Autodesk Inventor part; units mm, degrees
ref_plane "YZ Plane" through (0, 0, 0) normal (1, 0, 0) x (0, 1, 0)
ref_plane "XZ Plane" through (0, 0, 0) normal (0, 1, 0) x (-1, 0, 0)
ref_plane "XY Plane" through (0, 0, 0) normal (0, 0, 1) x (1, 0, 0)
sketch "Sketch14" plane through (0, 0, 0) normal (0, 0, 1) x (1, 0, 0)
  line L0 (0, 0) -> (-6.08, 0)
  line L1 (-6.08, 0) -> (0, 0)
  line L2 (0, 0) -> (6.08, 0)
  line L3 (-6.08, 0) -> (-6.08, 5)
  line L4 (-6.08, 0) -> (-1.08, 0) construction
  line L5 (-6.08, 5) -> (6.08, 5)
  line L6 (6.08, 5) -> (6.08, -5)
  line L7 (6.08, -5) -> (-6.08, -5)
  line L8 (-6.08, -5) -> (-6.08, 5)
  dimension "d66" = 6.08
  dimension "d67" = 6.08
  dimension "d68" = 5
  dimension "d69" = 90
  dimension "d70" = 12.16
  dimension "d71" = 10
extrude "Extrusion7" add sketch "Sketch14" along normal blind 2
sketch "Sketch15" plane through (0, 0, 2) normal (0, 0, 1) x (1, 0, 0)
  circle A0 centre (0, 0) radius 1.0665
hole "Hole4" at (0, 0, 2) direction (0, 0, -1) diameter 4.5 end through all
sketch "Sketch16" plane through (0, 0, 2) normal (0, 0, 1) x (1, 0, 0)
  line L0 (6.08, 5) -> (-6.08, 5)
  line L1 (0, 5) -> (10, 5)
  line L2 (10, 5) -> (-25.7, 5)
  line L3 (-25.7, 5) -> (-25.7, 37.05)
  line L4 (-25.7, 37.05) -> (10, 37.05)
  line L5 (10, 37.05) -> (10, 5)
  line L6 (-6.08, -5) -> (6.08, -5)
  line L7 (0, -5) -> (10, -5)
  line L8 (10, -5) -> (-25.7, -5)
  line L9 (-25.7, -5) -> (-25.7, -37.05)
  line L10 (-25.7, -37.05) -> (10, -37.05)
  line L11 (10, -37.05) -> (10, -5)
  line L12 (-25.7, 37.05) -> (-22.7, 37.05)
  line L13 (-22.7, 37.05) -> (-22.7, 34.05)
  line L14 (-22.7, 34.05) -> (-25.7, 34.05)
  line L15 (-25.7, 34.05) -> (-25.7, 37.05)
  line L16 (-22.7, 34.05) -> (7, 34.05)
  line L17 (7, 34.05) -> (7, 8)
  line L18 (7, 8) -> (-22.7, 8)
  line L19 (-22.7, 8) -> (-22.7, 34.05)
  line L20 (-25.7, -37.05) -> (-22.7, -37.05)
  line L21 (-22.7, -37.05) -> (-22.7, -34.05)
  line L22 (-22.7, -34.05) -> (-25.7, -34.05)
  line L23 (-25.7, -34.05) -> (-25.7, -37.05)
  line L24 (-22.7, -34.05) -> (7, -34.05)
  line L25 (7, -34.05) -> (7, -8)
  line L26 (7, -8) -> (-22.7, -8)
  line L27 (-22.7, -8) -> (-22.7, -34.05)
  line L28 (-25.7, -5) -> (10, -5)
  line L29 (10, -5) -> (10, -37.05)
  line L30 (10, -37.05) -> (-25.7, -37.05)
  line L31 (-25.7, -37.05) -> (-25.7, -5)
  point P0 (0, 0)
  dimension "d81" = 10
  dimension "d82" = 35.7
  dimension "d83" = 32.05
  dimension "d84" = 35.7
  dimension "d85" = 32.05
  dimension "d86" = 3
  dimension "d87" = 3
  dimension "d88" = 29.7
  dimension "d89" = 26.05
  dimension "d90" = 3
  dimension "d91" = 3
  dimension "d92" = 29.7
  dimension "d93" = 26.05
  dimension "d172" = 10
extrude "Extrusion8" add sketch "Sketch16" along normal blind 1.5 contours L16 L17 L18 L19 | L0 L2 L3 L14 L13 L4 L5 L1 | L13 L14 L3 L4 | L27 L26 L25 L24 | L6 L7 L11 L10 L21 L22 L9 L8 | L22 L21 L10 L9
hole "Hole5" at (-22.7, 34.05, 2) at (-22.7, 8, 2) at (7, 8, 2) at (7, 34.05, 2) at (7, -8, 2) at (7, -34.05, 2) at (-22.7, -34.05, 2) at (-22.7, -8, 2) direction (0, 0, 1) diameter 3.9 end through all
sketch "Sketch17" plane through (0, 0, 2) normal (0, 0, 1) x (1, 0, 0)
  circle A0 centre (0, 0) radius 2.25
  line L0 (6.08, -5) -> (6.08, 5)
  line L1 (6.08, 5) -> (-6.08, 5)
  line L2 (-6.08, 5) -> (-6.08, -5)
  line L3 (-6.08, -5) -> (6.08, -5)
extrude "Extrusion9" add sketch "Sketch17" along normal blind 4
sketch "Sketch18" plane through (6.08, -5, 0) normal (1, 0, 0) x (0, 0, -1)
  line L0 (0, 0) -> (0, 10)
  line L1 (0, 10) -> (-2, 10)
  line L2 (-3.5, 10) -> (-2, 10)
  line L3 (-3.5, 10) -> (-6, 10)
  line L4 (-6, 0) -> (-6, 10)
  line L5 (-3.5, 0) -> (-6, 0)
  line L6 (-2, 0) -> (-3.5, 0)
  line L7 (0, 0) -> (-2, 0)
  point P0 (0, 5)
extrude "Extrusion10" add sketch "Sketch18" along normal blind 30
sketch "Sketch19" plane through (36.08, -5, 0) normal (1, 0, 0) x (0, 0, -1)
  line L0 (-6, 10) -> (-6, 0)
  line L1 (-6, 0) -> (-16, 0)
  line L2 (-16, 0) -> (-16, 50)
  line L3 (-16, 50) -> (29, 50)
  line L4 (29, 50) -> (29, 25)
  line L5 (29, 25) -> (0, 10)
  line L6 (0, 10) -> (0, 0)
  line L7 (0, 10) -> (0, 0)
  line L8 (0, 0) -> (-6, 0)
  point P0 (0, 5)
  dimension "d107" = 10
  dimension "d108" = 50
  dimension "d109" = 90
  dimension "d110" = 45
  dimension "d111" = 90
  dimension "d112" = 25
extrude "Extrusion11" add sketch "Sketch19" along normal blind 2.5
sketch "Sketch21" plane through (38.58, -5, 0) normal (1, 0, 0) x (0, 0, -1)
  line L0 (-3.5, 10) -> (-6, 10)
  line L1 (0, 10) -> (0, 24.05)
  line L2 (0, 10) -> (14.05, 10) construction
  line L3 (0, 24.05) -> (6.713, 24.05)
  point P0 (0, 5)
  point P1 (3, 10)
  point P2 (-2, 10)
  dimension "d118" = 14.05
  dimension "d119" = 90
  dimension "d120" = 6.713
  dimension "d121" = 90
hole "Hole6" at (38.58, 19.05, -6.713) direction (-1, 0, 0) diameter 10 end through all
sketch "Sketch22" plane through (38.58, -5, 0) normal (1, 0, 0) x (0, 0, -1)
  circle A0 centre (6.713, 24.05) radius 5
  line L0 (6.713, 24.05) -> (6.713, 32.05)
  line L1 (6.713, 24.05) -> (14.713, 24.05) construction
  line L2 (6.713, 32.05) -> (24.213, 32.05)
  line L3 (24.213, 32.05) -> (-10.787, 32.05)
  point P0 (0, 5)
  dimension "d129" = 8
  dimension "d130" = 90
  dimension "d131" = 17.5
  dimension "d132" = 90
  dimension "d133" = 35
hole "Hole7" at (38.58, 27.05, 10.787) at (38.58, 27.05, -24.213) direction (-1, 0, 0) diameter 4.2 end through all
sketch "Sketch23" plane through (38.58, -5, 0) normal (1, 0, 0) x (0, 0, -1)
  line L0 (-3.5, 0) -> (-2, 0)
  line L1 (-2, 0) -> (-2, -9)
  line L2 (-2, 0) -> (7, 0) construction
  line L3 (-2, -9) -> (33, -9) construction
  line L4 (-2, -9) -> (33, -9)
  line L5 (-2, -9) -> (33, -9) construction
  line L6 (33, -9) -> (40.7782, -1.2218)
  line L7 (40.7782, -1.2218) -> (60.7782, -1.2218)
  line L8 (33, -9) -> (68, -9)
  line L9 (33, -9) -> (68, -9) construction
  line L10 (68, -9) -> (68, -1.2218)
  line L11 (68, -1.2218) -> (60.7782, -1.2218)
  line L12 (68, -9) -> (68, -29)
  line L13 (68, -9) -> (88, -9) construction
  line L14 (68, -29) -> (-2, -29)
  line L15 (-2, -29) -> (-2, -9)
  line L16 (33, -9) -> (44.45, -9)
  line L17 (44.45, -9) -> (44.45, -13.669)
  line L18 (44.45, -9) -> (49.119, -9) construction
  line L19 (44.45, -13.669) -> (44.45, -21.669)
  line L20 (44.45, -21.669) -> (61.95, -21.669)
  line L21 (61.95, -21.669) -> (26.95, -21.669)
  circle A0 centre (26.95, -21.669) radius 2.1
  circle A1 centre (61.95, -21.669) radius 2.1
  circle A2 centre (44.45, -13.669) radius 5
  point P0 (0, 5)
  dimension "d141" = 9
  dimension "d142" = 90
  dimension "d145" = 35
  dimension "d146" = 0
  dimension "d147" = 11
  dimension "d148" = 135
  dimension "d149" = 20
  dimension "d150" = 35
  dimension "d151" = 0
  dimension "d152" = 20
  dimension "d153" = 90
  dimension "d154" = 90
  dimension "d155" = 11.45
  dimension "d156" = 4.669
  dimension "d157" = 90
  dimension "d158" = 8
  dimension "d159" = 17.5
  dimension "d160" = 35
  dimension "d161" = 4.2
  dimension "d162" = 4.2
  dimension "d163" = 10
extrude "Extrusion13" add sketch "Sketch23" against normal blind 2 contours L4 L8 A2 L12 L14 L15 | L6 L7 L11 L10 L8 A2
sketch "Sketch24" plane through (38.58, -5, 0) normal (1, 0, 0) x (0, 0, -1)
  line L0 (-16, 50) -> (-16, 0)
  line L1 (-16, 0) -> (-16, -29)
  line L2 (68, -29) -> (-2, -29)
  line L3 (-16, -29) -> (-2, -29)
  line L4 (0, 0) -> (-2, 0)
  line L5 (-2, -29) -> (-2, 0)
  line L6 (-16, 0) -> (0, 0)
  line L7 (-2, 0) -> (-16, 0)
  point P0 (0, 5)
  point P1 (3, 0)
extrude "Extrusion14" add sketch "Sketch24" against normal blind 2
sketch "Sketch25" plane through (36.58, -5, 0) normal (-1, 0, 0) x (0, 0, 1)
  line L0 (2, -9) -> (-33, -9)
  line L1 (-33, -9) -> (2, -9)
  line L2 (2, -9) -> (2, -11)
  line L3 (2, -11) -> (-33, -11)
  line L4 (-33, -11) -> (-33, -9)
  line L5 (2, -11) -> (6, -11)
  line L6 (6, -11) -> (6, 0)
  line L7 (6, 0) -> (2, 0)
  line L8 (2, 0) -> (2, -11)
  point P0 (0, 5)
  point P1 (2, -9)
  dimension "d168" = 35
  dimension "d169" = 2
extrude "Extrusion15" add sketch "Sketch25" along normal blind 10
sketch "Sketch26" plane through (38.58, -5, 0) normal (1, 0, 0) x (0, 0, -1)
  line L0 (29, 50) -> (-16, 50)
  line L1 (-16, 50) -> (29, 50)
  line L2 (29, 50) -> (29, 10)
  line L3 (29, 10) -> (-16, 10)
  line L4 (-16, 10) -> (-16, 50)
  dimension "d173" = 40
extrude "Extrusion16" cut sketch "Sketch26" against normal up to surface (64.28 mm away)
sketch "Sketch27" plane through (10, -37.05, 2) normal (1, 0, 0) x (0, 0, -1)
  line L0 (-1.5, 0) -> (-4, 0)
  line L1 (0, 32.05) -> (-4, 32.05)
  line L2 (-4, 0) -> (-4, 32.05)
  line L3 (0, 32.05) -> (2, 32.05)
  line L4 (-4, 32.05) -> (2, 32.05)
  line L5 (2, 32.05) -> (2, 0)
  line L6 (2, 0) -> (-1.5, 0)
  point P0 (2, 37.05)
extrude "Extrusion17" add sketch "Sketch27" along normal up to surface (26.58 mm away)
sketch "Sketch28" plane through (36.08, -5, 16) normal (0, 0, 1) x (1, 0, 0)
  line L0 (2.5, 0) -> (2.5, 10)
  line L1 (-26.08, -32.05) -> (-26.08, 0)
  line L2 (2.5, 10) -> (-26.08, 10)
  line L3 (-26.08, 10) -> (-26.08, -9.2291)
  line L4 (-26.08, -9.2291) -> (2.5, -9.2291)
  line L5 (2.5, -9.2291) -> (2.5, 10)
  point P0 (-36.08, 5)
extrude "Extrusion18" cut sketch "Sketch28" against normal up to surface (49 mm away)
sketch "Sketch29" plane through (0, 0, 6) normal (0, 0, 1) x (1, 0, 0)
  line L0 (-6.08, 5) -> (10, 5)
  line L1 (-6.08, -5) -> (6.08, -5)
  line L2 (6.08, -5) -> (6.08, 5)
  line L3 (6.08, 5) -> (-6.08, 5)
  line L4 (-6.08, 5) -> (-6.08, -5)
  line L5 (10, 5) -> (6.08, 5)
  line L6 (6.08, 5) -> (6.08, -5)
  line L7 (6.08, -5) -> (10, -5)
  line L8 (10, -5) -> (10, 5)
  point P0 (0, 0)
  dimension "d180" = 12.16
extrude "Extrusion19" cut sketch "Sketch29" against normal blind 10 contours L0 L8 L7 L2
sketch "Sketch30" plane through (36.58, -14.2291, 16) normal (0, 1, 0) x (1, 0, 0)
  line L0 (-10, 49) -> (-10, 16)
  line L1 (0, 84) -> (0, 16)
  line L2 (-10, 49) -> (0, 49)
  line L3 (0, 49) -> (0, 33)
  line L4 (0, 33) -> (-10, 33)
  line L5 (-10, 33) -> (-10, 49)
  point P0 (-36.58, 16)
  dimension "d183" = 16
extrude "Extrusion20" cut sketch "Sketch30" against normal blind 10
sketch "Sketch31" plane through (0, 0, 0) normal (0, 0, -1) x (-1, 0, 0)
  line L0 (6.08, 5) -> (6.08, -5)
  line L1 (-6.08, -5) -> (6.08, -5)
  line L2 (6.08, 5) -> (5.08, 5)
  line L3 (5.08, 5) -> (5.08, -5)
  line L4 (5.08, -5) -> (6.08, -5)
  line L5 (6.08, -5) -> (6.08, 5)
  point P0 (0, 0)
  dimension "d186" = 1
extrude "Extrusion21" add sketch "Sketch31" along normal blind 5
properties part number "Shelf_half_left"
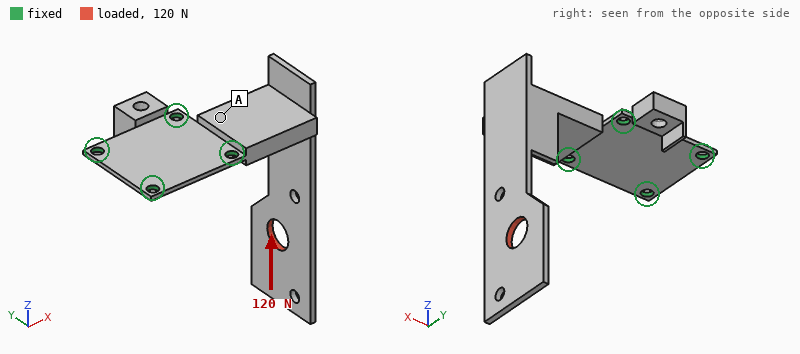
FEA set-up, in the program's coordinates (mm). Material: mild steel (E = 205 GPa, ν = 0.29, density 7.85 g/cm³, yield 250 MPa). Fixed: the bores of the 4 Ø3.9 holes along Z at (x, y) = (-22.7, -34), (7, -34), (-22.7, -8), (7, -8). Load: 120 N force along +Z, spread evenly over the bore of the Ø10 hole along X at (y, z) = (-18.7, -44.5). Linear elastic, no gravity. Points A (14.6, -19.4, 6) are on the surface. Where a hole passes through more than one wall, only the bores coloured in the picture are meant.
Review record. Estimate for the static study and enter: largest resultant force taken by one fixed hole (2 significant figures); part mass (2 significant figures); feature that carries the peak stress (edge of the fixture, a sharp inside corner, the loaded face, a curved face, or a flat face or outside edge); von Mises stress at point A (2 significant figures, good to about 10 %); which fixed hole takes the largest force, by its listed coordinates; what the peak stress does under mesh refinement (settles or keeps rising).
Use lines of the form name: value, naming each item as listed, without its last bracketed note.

largest resultant force taken by one fixed hole: 92 N
part mass: 78 g
feature that carries the peak stress: edge of the fixture
von Mises stress at point A: 27 MPa
which fixed hole takes the largest force, by its listed coordinates: (7, -8)
what the peak stress does under mesh refinement: keeps rising
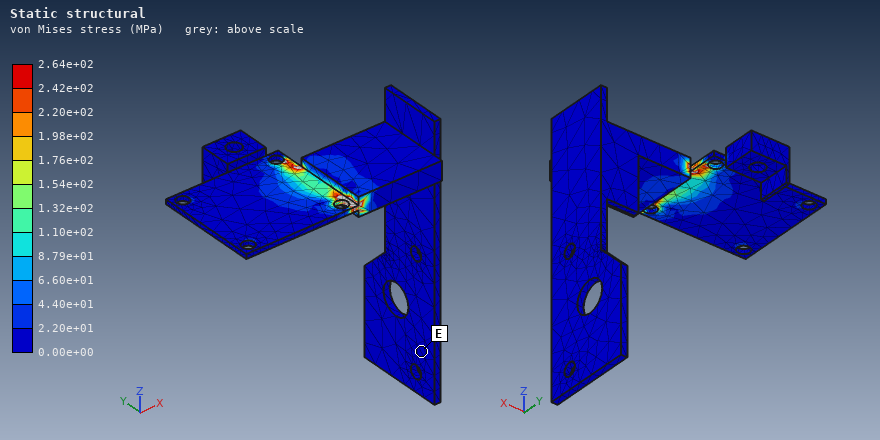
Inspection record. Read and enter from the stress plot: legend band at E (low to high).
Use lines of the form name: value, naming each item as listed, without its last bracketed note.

legend band at E: 0.00e+00 to 2.20e+01 MPa
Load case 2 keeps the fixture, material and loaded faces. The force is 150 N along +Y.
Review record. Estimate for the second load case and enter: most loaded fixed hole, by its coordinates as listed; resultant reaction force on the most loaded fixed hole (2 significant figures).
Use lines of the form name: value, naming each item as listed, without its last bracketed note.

most loaded fixed hole, by its coordinates as listed: (7, -34)
resultant reaction force on the most loaded fixed hole: 360 N
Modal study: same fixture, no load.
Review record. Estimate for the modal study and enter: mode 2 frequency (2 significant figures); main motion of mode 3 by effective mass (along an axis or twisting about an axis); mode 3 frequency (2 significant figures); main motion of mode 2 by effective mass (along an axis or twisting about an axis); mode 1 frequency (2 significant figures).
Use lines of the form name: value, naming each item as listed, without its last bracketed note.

mode 2 frequency: 750 Hz
main motion of mode 3 by effective mass: along Y
mode 3 frequency: 1000 Hz
main motion of mode 2 by effective mass: along Z
mode 1 frequency: 290 Hz
